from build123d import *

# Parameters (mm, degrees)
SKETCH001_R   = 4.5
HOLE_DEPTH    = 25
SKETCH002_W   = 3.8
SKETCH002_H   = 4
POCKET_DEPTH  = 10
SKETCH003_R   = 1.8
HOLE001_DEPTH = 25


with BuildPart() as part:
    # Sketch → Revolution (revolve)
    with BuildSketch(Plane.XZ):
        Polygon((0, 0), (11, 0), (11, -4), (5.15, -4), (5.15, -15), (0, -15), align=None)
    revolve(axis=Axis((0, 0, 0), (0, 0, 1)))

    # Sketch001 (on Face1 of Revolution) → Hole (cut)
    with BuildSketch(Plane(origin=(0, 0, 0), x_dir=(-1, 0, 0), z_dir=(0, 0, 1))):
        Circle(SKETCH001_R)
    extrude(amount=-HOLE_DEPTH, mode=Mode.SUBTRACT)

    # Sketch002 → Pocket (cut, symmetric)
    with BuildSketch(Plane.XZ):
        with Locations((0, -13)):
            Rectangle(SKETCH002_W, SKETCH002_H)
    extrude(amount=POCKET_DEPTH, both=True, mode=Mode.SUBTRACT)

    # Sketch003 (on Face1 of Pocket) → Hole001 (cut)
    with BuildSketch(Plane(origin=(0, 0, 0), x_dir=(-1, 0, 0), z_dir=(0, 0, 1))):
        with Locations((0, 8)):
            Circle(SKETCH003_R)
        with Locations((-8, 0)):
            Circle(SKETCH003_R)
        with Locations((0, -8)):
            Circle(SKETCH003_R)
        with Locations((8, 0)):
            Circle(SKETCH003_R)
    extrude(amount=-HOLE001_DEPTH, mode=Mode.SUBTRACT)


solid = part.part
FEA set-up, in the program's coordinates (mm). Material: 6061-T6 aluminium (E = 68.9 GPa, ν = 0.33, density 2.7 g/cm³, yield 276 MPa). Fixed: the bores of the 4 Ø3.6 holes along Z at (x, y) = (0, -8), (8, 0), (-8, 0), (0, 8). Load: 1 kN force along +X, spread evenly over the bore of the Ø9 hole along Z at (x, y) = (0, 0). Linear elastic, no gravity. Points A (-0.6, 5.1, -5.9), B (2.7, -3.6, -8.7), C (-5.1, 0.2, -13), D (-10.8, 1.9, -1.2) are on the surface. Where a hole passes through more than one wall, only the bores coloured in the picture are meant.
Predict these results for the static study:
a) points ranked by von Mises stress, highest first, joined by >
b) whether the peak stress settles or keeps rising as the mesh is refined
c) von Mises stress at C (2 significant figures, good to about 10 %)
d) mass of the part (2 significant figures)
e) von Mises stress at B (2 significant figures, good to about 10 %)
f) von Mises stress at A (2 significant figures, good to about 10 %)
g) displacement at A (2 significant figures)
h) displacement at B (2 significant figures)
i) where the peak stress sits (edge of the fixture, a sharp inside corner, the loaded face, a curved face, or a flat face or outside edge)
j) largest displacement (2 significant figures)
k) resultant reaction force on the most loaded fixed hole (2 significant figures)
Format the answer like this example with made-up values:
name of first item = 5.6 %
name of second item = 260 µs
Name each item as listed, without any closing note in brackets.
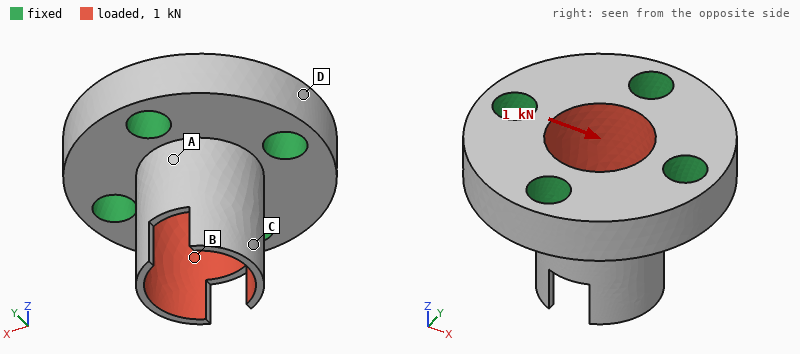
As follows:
points ranked by von Mises stress, highest first, joined by > = A > B > C > D
whether the peak stress settles or keeps rising as the mesh is refined = keeps rising
von Mises stress at C = 32 MPa
mass of the part = 3.5 g
von Mises stress at B = 64 MPa
von Mises stress at A = 96 MPa
displacement at A = 6.9 µm
displacement at B = 14 µm
where the peak stress sits = a sharp inside corner
largest displacement = 42 µm
resultant reaction force on the most loaded fixed hole = 440 N
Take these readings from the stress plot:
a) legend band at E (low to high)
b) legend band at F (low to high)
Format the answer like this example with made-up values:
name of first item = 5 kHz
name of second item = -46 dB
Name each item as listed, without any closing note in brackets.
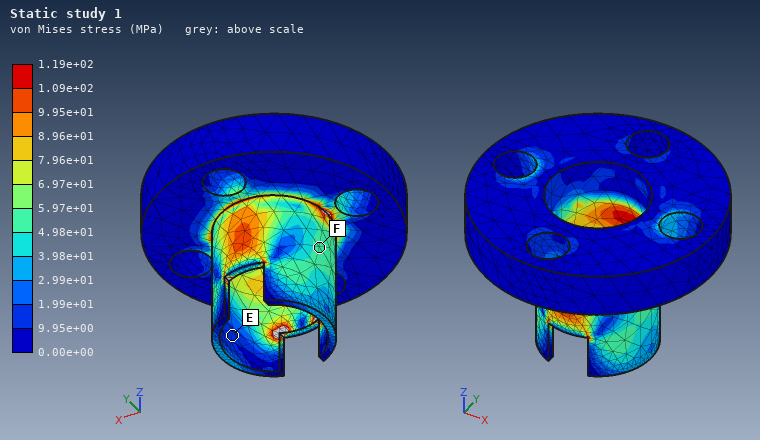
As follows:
legend band at E = 9.95e+00 to 1.99e+01 MPa
legend band at F = 4.98e+01 to 5.97e+01 MPa
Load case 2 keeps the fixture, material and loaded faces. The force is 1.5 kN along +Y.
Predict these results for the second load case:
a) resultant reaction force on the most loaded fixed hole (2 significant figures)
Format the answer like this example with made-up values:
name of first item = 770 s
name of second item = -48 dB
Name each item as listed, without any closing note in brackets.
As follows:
resultant reaction force on the most loaded fixed hole = 660 N
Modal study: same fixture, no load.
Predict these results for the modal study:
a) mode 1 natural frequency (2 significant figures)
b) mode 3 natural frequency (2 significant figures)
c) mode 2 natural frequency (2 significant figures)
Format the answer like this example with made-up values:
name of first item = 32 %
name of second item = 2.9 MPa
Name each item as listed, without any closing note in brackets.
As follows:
mode 1 natural frequency = 22 kHz
mode 3 natural frequency = 28 kHz
mode 2 natural frequency = 27 kHz
